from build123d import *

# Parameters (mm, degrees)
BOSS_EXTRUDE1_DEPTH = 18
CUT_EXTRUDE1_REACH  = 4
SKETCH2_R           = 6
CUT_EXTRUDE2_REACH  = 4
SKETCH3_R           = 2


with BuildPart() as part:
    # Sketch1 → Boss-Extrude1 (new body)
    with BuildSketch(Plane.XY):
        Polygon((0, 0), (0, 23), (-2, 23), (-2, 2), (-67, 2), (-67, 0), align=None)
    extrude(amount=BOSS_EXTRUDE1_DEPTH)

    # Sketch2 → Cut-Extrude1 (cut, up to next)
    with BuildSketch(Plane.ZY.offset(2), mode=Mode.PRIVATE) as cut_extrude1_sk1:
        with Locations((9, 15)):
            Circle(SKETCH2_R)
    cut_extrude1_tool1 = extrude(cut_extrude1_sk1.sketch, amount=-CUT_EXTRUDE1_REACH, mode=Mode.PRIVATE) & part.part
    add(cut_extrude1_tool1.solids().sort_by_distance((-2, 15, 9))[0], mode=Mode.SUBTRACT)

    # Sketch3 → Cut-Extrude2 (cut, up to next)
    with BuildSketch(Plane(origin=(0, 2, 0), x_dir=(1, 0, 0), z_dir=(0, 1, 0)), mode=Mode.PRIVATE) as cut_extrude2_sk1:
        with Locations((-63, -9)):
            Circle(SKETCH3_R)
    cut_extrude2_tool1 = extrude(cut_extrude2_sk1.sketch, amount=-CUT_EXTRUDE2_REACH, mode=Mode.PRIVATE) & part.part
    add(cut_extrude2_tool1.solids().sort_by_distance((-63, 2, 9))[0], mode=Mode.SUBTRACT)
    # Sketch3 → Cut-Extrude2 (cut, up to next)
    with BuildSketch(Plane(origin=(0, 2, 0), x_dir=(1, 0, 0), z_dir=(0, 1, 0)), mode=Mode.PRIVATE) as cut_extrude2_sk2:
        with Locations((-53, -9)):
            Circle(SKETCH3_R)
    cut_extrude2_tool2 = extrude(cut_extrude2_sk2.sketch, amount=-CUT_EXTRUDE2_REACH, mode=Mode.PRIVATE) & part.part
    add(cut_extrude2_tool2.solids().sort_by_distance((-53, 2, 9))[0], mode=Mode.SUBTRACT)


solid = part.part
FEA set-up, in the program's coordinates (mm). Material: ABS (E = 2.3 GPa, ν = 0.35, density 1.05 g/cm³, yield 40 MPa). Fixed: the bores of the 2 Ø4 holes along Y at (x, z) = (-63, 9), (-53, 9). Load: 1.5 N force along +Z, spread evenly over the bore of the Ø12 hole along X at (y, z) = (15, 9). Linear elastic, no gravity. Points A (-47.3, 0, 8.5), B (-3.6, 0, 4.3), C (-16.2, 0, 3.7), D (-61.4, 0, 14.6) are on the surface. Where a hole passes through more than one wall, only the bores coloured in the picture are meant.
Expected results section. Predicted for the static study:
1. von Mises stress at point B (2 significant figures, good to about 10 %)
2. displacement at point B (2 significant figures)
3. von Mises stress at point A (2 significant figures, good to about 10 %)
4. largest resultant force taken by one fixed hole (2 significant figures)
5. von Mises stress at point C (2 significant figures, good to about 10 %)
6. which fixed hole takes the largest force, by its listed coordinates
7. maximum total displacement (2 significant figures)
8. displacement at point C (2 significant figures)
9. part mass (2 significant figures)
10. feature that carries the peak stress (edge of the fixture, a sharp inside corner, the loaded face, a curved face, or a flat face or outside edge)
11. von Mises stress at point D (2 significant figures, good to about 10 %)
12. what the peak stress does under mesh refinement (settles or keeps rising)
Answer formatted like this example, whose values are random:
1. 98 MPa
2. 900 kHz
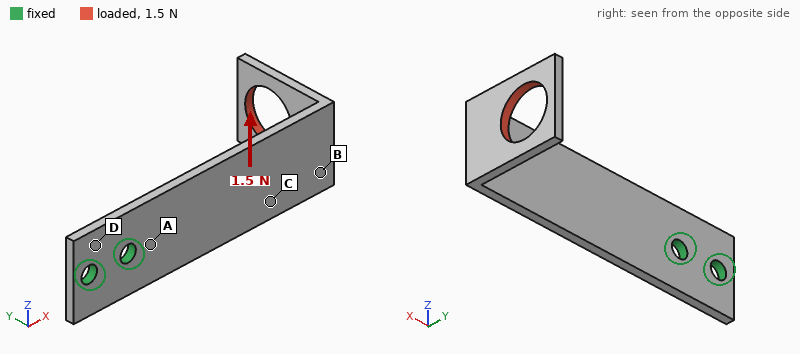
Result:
1. 1.1 MPa
2. 0.12 mm
3. 1.4 MPa
4. 6.1 N
5. 1.5 MPa
6. (-53, 9)
7. 0.68 mm
8. 0.10 mm
9. 3.0 g
10. edge of the fixture
11. 0.37 MPa
12. keeps rising
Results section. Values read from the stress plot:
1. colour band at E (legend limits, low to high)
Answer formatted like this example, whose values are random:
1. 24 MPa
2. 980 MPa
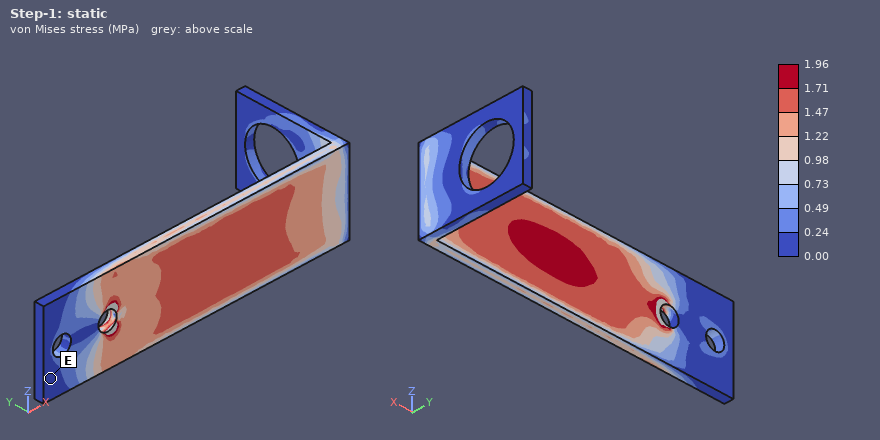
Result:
1. 0.00 to 0.24 MPa
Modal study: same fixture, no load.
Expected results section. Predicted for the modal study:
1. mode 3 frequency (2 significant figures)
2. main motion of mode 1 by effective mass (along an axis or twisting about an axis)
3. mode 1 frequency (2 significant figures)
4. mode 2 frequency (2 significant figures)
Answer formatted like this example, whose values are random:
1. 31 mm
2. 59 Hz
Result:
1. 570 Hz
2. along Y
3. 120 Hz
4. 390 Hz
